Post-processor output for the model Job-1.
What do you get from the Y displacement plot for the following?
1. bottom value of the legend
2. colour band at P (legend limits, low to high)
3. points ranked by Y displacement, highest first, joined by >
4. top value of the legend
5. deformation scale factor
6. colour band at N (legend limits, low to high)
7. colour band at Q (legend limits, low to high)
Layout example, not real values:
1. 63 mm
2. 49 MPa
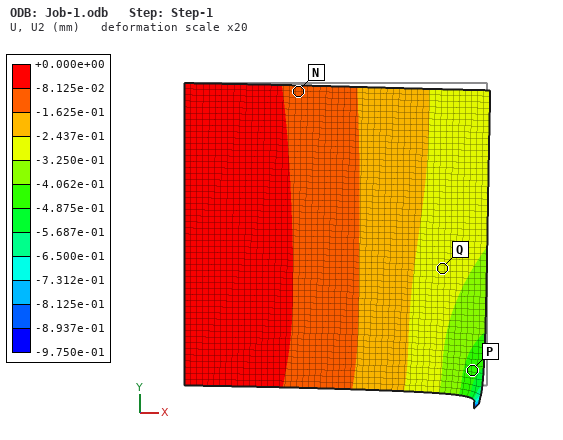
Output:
1. -9.750e-01 mm
2. -4.875e-01 to -4.062e-01 mm
3. N > Q > P
4. +0.000e+00 mm
5. 20
6. -1.625e-01 to -8.125e-02 mm
7. -3.250e-01 to -2.437e-01 mm
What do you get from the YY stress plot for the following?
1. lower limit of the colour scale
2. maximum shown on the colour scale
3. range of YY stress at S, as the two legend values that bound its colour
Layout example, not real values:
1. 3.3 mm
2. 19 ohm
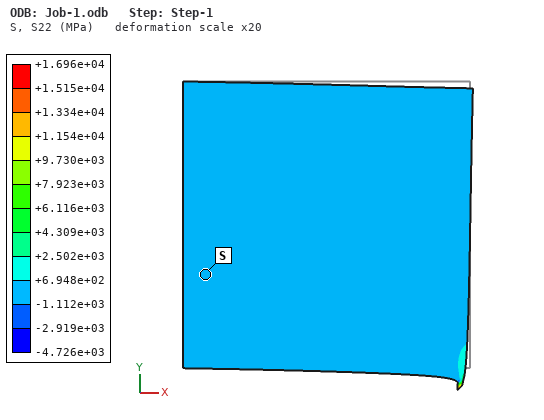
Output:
1. -4.726e+03 MPa
2. +1.696e+04 MPa
3. -1.112e+03 to +6.948e+02 MPa
